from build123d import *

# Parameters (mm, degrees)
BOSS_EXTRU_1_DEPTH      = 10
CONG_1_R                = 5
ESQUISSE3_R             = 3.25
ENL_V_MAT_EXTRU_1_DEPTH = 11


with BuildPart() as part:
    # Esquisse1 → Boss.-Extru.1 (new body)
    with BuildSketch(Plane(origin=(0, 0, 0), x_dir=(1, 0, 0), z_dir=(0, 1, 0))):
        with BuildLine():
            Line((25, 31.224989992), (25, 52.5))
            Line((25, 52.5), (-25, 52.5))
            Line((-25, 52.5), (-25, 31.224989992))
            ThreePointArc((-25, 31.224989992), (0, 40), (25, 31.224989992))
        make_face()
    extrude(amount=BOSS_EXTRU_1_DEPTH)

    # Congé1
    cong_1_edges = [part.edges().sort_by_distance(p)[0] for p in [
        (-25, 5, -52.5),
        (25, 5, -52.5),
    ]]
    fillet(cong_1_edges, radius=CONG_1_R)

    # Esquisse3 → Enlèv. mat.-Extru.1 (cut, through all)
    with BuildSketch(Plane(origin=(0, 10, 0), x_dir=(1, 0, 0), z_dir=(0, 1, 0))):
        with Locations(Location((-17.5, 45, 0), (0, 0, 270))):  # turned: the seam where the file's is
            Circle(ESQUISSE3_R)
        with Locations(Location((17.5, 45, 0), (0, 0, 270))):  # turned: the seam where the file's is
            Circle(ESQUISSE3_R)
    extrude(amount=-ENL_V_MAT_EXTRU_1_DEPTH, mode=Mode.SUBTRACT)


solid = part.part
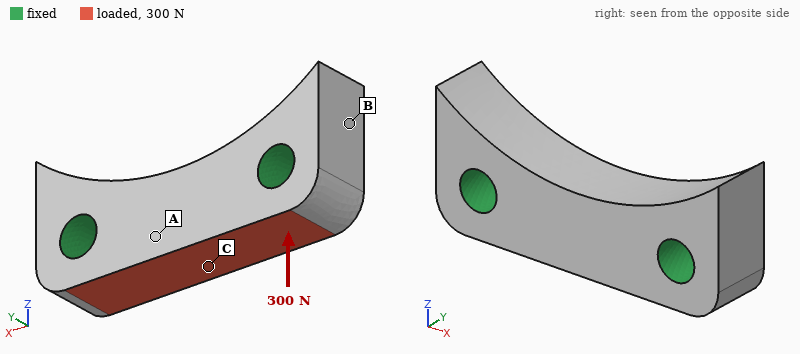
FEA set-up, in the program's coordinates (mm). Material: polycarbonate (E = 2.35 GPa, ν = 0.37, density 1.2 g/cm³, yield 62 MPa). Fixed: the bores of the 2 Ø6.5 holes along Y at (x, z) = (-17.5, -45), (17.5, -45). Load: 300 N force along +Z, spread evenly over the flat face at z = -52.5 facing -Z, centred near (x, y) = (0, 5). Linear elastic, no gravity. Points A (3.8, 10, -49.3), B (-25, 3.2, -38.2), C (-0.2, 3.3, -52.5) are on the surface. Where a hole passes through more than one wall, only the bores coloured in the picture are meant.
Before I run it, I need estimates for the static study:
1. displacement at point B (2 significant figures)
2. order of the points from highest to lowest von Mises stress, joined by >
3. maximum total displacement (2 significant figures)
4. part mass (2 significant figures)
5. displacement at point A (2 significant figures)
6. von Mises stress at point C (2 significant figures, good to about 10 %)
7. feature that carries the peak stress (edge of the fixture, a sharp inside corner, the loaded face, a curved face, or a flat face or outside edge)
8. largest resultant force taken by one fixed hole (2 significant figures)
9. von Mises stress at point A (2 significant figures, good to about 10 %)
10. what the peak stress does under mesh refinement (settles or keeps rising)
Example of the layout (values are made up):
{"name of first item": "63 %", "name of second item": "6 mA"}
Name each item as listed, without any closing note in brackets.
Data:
{"displacement at point B": "3.1 µm", "order of the points from highest to lowest von Mises stress, joined by >": "C > A > B", "maximum total displacement": "17 µm", "part mass": "8.2 g", "displacement at point A": "15 µm", "von Mises stress at point C": "1.7 MPa", "feature that carries the peak stress": "edge of the fixture", "largest resultant force taken by one fixed hole": "150 N", "von Mises stress at point A": "0.90 MPa", "what the peak stress does under mesh refinement": "keeps rising"}
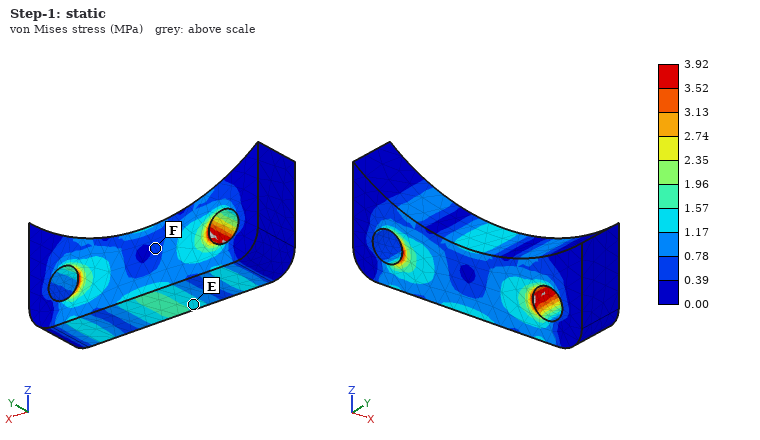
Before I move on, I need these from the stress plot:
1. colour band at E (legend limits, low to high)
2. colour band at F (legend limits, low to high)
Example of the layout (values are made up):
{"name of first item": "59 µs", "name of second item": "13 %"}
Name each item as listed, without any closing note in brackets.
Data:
{"colour band at E": "1.17 to 1.57 MPa", "colour band at F": "0.39 to 0.78 MPa"}
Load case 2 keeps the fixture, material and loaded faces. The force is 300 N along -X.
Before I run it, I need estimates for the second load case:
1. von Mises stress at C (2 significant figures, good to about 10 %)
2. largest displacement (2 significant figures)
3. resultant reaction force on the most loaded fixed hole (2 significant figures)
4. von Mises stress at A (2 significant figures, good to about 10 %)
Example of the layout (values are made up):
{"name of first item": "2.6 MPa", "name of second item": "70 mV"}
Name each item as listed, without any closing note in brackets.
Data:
{"von Mises stress at C": "1.3 MPa", "largest displacement": "7.4 µm", "resultant reaction force on the most loaded fixed hole": "160 N", "von Mises stress at A": "1.0 MPa"}
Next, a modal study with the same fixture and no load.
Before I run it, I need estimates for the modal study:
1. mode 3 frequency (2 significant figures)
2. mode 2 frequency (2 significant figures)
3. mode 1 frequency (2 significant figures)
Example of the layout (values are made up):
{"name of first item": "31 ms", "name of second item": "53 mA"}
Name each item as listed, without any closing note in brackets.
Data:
{"mode 3 frequency": "13 kHz", "mode 2 frequency": "9700 Hz", "mode 1 frequency": "9700 Hz"}
